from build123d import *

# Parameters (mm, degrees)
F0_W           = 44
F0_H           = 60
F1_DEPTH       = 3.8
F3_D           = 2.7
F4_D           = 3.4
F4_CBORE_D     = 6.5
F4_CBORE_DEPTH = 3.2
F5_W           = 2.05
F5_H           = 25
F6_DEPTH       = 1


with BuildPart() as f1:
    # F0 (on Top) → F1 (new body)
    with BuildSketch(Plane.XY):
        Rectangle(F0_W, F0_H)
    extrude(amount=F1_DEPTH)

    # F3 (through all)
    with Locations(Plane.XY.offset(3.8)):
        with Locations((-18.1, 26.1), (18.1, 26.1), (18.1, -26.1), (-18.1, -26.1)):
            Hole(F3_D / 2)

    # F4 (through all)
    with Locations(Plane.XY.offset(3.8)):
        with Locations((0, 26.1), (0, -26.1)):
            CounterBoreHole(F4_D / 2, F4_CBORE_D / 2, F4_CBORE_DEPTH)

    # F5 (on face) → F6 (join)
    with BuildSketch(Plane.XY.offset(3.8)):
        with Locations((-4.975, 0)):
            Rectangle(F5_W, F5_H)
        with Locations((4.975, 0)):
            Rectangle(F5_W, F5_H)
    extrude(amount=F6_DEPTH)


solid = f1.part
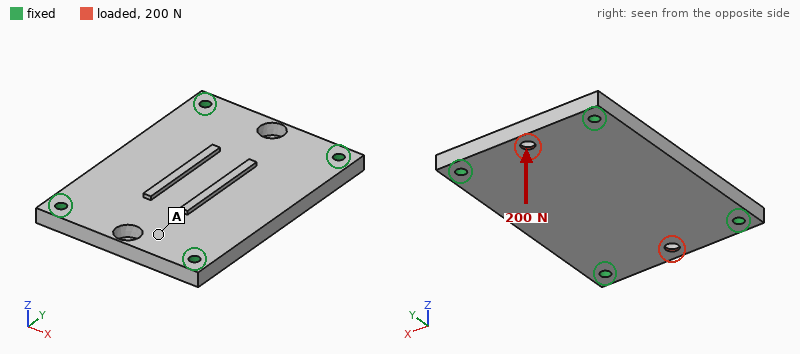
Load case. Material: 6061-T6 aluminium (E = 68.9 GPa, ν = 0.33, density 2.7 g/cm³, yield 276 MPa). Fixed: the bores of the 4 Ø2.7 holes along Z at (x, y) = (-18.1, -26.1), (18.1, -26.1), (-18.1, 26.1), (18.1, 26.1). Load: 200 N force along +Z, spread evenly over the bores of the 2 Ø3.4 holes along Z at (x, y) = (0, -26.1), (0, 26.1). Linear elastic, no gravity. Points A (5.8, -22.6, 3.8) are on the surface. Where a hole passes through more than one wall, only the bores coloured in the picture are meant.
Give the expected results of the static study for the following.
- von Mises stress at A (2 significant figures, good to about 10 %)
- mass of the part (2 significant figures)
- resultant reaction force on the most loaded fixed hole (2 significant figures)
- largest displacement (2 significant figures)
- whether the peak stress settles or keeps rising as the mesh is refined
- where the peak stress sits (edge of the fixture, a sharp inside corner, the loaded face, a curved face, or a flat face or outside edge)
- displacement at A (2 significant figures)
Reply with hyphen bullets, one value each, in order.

- 8.4 MPa
- 27 g
- 53 N
- 17 µm
- keeps rising
- a sharp inside corner
- 5.1 µm
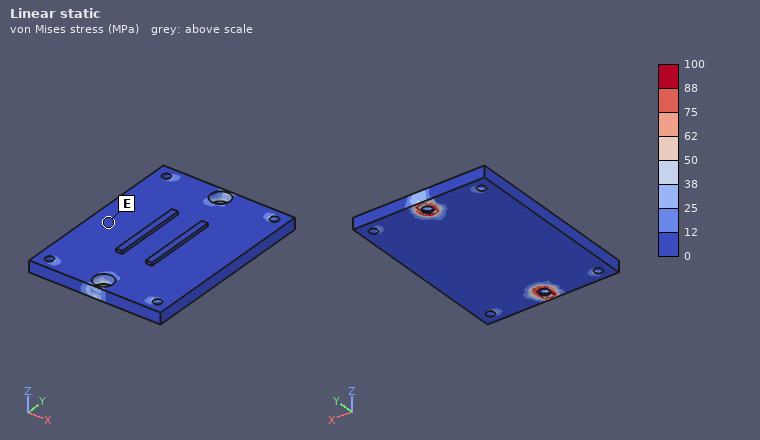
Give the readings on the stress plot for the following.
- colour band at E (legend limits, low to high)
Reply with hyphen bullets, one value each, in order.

- 0 to 12 MPa
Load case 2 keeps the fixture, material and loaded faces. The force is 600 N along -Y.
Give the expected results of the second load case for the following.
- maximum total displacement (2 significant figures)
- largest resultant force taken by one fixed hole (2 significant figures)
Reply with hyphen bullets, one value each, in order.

- 7.5 µm
- 160 N
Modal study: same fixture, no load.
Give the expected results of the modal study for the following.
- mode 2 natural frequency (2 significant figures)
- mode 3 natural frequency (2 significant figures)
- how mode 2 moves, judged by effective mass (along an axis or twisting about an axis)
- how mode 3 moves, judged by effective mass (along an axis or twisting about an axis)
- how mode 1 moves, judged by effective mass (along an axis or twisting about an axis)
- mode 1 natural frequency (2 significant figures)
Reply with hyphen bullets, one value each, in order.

- 8700 Hz
- 13 kHz
- twisting about Y
- twisting about X
- along Z
- 5700 Hz
